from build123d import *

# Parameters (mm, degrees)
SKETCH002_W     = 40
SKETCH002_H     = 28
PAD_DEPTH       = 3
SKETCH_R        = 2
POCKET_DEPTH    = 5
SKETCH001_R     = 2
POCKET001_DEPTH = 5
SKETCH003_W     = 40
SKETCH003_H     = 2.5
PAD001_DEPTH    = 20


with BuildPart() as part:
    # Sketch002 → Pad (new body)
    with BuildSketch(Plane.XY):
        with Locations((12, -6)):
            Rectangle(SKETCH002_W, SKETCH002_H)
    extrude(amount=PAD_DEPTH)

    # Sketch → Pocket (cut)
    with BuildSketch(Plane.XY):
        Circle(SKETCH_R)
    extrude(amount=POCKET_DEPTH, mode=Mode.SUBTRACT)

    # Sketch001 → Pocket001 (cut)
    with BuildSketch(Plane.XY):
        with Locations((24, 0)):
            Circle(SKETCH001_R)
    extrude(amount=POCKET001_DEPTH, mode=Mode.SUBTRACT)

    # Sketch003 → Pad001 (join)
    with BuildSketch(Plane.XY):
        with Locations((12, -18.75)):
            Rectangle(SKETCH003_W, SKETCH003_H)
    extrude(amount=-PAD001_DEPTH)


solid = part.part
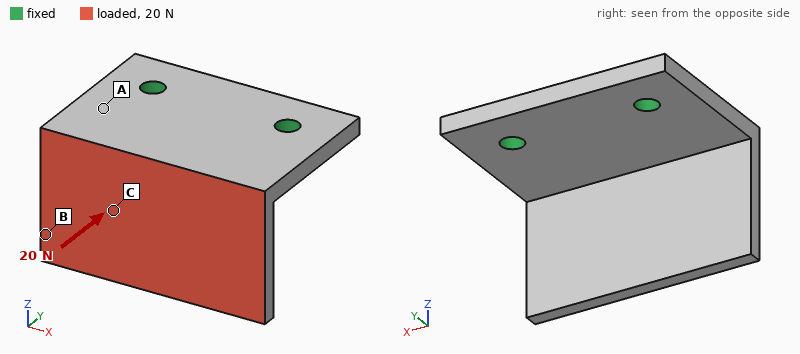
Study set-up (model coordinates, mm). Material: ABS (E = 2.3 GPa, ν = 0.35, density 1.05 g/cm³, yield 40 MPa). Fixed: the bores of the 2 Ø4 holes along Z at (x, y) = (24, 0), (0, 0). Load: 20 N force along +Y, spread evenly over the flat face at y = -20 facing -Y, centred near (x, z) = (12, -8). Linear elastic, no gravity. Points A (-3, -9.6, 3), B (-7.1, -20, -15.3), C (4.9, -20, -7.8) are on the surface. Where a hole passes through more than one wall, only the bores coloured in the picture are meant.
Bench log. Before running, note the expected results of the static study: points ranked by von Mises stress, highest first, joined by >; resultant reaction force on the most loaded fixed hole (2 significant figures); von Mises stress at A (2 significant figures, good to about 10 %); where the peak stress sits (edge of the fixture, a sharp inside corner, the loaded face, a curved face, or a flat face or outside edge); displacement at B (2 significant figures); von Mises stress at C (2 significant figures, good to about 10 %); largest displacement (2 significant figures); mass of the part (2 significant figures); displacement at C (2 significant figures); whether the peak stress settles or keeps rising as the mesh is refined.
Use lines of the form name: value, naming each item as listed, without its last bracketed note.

points ranked by von Mises stress, highest first, joined by >: A > C > B
resultant reaction force on the most loaded fixed hole: 10 N
von Mises stress at A: 3.0 MPa
where the peak stress sits: edge of the fixture
displacement at B: 0.43 mm
von Mises stress at C: 1.4 MPa
largest displacement: 0.54 mm
mass of the part: 5.5 g
displacement at C: 0.27 mm
whether the peak stress settles or keeps rising as the mesh is refined: keeps rising
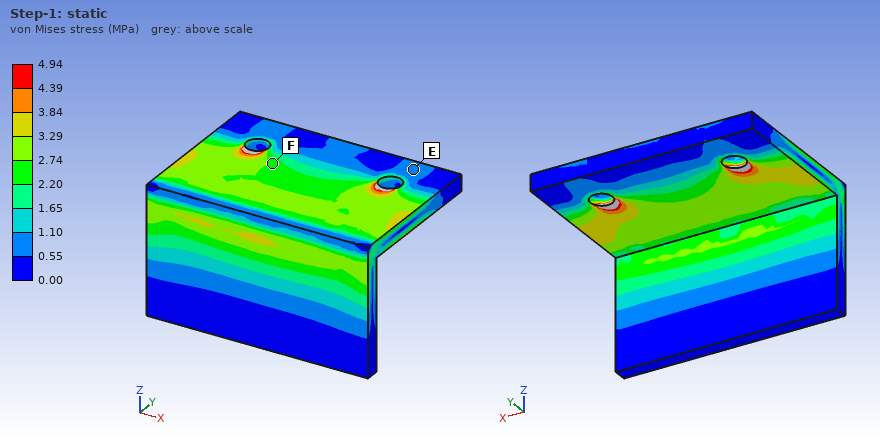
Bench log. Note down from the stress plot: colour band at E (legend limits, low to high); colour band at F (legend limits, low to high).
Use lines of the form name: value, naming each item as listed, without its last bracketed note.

colour band at E: 0.55 to 1.10 MPa
colour band at F: 2.20 to 2.74 MPa
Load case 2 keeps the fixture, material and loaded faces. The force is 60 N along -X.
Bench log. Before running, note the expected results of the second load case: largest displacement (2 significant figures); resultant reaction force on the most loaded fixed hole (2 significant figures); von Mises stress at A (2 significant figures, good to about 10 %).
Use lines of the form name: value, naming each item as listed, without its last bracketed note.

largest displacement: 0.46 mm
resultant reaction force on the most loaded fixed hole: 58 N
von Mises stress at A: 3.8 MPa
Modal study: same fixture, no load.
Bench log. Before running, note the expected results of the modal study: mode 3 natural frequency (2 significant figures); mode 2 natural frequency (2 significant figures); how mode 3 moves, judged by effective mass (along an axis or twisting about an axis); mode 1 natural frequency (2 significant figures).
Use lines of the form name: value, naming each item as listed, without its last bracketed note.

mode 3 natural frequency: 1600 Hz
mode 2 natural frequency: 1100 Hz
how mode 3 moves, judged by effective mass: along Z
mode 1 natural frequency: 650 Hz
